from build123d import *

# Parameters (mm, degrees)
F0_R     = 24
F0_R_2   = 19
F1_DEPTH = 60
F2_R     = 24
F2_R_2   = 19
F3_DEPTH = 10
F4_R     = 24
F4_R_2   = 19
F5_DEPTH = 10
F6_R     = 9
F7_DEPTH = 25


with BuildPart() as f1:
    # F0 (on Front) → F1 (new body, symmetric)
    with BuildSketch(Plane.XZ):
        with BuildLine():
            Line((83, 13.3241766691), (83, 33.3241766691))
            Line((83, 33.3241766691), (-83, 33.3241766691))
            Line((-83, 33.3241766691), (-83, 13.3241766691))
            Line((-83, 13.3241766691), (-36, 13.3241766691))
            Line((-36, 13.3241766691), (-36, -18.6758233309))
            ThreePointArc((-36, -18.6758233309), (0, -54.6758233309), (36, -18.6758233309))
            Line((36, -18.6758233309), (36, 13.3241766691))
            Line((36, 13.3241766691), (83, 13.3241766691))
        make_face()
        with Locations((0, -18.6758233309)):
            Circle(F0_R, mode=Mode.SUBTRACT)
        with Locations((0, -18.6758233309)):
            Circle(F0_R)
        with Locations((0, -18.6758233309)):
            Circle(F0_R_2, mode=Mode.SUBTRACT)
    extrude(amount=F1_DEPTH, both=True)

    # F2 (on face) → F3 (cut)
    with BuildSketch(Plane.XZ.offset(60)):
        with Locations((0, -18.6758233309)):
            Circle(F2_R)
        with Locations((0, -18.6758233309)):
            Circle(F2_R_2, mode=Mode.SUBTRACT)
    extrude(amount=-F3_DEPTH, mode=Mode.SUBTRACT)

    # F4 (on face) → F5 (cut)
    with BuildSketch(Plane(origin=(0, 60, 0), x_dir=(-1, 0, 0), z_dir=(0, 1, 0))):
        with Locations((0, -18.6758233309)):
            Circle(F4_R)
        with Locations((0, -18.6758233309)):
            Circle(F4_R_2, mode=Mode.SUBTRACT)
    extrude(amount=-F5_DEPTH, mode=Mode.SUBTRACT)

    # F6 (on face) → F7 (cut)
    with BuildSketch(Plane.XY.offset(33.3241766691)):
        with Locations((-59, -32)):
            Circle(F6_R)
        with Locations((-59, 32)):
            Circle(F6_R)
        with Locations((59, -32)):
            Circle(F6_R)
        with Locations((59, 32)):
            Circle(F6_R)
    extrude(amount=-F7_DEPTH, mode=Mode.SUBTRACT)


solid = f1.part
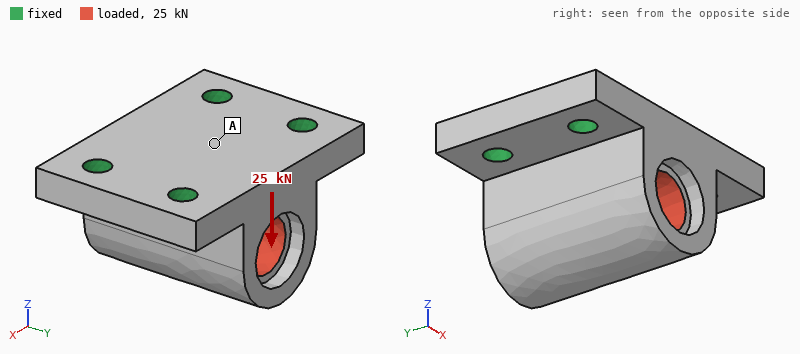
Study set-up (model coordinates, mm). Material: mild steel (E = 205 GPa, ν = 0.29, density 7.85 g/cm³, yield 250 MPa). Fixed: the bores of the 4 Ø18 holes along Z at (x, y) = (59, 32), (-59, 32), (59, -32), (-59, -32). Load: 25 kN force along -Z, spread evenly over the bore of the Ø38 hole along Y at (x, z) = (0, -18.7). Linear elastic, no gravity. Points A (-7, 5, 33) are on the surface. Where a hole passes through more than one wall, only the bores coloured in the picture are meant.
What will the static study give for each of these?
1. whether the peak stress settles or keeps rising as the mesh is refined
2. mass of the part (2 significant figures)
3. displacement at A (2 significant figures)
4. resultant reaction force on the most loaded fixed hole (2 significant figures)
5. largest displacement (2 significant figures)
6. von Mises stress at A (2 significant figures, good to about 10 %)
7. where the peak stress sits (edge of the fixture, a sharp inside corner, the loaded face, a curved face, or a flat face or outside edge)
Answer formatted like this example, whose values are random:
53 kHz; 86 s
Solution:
keeps rising; 5.9 kg; 4.7 µm; 6.7 kN; 5.5 µm; 5.6 MPa; edge of the fixture
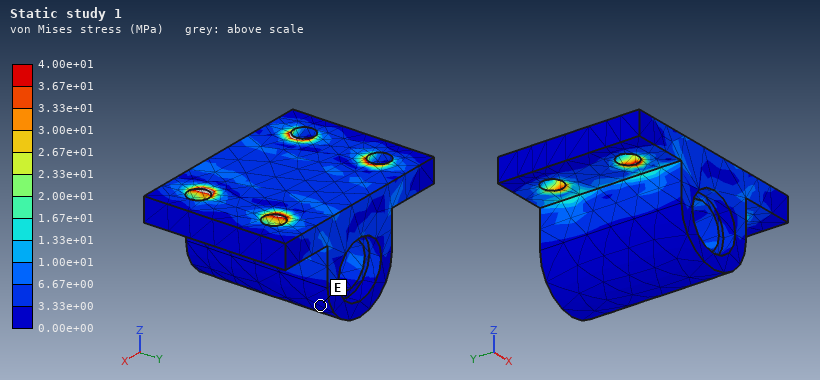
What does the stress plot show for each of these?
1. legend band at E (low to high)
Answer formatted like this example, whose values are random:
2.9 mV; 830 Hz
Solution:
0.00e+00 to 3.33e+00 MPa
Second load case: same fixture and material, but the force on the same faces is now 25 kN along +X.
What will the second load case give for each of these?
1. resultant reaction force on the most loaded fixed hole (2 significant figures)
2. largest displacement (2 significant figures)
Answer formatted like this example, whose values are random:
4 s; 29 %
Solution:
8.5 kN; 12 µm
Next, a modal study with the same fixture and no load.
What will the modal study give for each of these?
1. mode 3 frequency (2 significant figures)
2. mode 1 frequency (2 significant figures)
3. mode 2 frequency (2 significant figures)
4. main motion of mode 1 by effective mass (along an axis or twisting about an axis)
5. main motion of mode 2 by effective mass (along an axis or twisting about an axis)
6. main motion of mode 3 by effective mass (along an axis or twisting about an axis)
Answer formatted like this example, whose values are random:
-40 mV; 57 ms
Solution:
5700 Hz; 3800 Hz; 4800 Hz; along Y; along X; along Z
